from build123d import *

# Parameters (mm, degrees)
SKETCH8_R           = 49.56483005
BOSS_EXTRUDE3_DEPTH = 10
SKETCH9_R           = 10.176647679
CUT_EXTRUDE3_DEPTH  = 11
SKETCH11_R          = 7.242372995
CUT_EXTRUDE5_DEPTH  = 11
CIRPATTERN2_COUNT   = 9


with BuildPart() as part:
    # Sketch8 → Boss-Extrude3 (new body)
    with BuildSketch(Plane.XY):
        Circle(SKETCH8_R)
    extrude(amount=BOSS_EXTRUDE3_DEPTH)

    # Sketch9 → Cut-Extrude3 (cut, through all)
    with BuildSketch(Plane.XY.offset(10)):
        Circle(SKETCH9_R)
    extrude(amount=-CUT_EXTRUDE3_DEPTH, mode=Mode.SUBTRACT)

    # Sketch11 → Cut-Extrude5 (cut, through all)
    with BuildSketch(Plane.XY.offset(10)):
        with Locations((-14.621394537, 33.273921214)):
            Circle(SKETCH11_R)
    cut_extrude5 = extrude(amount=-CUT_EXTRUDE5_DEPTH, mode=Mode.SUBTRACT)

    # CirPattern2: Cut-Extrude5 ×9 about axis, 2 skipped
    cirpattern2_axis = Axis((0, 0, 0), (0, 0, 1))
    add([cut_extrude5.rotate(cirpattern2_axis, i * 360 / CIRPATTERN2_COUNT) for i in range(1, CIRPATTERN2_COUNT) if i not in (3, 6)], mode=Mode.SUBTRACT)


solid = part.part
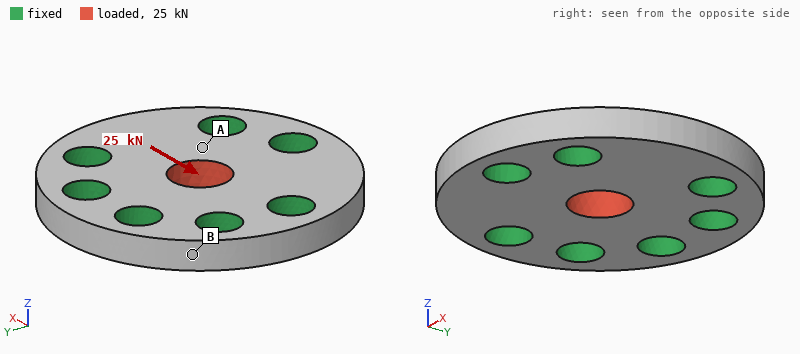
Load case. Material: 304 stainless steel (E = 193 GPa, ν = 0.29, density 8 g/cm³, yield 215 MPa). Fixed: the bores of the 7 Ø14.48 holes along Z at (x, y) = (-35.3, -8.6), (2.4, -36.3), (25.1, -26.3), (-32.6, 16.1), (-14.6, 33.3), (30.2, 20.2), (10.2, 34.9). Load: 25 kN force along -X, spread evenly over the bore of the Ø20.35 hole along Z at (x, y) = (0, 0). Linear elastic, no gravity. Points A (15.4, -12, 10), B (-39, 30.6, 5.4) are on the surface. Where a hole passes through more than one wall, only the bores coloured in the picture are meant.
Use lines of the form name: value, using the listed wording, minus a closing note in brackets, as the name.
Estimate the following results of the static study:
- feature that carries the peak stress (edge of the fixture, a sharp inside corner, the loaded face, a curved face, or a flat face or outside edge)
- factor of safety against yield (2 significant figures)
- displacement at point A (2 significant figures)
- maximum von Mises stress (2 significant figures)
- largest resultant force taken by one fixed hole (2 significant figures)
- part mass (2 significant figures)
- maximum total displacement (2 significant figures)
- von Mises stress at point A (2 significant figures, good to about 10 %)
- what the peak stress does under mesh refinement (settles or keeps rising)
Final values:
feature that carries the peak stress: the loaded face
factor of safety against yield: 3.2
displacement at point A: 2.2 µm
maximum von Mises stress: 68 MPa
largest resultant force taken by one fixed hole: 6.2 kN
part mass: 500 g
maximum total displacement: 4.5 µm
von Mises stress at point A: 30 MPa
what the peak stress does under mesh refinement: settles
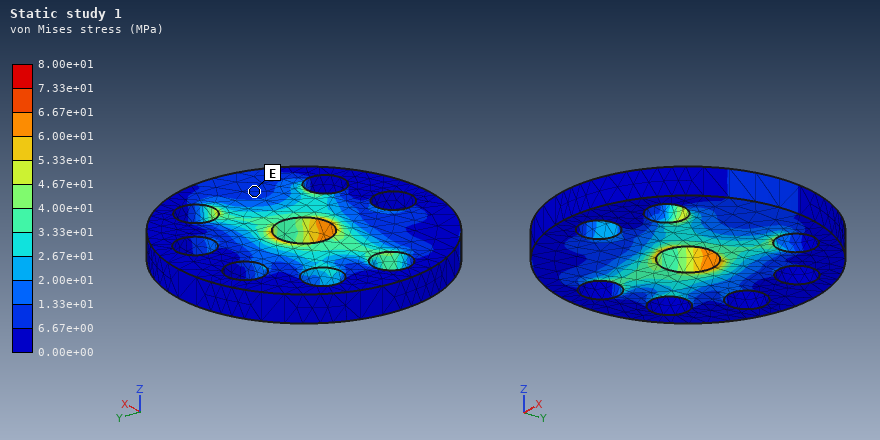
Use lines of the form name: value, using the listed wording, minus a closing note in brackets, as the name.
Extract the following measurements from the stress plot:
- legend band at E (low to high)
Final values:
legend band at E: 6.67e+00 to 1.33e+01 MPa
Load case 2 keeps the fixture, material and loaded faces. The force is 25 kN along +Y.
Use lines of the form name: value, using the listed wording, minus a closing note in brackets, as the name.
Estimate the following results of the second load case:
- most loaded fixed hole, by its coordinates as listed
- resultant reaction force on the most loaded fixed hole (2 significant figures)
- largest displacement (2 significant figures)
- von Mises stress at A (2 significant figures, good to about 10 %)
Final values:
most loaded fixed hole, by its coordinates as listed: (2.4, -36.3)
resultant reaction force on the most loaded fixed hole: 6.4 kN
largest displacement: 4.2 µm
von Mises stress at A: 25 MPa
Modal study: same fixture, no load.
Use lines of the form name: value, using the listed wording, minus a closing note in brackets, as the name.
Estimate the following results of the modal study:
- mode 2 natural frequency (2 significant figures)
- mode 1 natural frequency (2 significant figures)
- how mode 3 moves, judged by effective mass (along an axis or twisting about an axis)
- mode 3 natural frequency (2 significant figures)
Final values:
mode 2 natural frequency: 19 kHz
mode 1 natural frequency: 18 kHz
how mode 3 moves, judged by effective mass: along Z
mode 3 natural frequency: 21 kHz
